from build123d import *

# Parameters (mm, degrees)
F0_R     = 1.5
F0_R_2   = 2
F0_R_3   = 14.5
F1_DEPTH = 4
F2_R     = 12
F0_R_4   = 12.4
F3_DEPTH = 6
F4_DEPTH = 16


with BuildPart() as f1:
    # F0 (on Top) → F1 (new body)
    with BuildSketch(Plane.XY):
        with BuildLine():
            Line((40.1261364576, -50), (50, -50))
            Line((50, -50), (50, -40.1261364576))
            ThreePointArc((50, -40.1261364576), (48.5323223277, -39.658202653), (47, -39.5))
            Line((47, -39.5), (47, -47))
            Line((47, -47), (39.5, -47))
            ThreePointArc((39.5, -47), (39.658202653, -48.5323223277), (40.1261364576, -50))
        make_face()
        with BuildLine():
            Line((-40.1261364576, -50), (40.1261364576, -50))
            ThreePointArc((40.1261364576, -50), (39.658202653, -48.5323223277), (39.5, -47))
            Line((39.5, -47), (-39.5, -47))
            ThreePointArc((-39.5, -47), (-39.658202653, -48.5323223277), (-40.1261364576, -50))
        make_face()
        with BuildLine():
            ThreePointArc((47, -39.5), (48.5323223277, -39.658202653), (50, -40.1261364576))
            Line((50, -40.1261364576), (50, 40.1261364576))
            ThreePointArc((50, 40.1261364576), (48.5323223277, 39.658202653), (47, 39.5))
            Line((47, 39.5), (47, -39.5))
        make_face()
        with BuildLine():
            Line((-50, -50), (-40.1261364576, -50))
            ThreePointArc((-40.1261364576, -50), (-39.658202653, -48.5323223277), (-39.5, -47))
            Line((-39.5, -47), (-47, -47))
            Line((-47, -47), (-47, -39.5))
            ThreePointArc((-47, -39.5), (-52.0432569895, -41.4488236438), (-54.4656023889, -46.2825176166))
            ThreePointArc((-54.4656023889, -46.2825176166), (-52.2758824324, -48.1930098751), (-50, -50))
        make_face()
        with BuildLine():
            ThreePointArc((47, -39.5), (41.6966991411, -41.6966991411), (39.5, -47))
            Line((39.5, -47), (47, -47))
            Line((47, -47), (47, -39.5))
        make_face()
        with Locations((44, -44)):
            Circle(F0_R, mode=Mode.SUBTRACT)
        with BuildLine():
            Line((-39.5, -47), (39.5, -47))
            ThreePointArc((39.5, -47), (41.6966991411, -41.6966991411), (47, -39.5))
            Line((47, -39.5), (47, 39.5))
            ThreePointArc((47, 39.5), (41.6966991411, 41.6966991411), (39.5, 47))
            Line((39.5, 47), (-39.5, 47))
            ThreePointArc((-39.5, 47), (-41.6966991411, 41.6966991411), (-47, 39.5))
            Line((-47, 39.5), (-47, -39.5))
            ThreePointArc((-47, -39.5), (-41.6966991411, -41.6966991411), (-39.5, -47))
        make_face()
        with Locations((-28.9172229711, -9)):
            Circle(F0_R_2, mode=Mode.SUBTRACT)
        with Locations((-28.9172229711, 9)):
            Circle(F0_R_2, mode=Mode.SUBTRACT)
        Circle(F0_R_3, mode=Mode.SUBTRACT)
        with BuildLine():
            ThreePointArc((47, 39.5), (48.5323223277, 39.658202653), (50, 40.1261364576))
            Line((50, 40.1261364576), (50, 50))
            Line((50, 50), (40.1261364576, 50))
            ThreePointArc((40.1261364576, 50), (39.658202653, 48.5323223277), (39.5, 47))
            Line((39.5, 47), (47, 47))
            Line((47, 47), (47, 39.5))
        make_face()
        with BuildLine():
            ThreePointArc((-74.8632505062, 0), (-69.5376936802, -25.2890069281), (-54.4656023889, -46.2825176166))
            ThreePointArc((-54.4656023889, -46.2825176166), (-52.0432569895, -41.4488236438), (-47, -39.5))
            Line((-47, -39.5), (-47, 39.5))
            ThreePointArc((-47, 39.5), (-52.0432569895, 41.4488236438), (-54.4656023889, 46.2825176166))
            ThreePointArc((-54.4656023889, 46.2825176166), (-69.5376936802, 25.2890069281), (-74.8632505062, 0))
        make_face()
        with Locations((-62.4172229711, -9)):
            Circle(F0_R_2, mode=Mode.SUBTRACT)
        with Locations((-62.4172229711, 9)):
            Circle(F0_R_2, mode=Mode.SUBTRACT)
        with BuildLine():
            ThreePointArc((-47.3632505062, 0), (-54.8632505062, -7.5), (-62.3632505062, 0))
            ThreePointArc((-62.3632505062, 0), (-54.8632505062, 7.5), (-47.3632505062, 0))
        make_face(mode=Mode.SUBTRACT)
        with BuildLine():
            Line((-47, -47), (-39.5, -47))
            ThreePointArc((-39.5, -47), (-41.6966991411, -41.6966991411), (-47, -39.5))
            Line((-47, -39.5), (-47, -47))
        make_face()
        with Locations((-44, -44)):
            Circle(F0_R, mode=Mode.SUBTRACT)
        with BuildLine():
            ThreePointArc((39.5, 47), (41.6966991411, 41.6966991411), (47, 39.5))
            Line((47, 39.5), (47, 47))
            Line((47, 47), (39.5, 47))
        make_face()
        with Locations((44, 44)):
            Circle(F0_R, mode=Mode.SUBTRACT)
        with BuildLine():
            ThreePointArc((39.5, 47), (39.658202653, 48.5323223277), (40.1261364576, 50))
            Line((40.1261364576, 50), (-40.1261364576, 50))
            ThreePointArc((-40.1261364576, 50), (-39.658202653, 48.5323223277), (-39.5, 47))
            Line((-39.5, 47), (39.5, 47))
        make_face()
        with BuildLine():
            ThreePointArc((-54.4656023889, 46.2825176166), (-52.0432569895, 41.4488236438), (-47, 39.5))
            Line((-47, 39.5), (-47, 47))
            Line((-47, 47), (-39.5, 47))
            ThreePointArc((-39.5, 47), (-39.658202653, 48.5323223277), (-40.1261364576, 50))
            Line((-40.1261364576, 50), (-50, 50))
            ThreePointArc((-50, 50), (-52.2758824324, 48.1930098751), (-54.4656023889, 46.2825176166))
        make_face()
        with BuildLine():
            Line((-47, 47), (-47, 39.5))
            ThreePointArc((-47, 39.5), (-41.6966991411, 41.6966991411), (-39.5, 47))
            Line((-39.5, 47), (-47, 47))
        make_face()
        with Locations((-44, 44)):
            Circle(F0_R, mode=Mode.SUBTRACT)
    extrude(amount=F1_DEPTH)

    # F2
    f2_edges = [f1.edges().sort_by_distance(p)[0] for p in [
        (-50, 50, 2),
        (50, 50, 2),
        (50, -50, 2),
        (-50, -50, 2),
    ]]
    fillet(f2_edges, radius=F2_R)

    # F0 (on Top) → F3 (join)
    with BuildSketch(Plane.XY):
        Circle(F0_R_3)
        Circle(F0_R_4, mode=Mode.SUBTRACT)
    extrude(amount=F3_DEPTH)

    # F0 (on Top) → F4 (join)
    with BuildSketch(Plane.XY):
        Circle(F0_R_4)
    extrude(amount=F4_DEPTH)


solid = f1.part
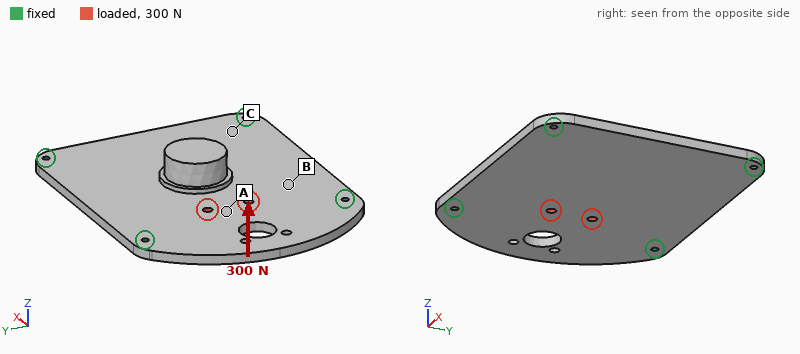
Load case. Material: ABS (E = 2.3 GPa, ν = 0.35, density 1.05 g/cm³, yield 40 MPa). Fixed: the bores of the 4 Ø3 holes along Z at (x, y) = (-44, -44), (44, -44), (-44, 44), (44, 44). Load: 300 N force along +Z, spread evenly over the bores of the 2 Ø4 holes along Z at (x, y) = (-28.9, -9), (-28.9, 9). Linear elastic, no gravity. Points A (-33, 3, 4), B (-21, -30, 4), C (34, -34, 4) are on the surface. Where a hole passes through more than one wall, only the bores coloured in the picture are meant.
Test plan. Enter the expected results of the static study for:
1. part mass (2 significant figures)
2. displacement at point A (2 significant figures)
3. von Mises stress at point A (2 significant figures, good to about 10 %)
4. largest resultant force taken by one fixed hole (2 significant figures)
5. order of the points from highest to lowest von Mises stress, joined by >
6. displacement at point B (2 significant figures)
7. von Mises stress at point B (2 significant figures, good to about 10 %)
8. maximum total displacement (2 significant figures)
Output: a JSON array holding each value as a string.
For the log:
["54 g", "1.9 mm", "17 MPa", "130 N", "A > B > C", "0.97 mm", "7.6 MPa", "1.9 mm"]
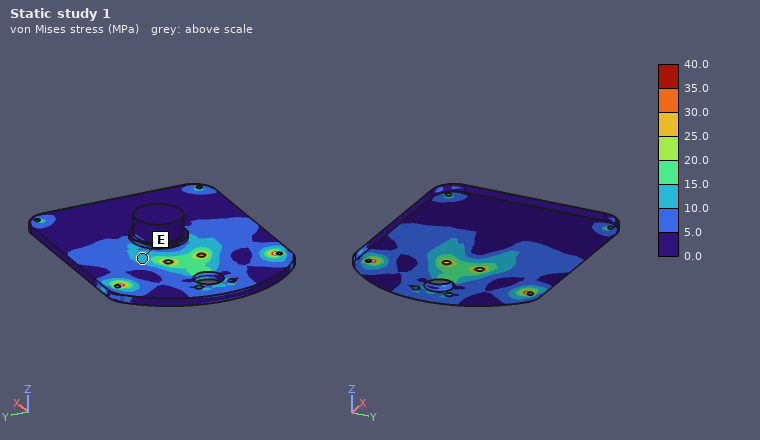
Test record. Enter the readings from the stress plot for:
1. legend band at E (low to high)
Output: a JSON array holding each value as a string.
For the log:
["10.0 to 15.0 MPa"]
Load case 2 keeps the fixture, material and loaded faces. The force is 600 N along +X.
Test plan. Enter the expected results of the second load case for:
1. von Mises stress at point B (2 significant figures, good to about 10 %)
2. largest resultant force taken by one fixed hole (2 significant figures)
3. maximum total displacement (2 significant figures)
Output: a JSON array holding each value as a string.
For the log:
["1.3 MPa", "180 N", "73 µm"]
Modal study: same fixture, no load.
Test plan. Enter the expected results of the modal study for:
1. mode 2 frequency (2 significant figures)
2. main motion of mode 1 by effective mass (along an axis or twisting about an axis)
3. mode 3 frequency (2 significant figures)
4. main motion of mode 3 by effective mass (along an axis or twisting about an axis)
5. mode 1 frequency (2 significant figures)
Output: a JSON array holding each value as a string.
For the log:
["580 Hz", "along Z", "800 Hz", "twisting about X", "430 Hz"]
